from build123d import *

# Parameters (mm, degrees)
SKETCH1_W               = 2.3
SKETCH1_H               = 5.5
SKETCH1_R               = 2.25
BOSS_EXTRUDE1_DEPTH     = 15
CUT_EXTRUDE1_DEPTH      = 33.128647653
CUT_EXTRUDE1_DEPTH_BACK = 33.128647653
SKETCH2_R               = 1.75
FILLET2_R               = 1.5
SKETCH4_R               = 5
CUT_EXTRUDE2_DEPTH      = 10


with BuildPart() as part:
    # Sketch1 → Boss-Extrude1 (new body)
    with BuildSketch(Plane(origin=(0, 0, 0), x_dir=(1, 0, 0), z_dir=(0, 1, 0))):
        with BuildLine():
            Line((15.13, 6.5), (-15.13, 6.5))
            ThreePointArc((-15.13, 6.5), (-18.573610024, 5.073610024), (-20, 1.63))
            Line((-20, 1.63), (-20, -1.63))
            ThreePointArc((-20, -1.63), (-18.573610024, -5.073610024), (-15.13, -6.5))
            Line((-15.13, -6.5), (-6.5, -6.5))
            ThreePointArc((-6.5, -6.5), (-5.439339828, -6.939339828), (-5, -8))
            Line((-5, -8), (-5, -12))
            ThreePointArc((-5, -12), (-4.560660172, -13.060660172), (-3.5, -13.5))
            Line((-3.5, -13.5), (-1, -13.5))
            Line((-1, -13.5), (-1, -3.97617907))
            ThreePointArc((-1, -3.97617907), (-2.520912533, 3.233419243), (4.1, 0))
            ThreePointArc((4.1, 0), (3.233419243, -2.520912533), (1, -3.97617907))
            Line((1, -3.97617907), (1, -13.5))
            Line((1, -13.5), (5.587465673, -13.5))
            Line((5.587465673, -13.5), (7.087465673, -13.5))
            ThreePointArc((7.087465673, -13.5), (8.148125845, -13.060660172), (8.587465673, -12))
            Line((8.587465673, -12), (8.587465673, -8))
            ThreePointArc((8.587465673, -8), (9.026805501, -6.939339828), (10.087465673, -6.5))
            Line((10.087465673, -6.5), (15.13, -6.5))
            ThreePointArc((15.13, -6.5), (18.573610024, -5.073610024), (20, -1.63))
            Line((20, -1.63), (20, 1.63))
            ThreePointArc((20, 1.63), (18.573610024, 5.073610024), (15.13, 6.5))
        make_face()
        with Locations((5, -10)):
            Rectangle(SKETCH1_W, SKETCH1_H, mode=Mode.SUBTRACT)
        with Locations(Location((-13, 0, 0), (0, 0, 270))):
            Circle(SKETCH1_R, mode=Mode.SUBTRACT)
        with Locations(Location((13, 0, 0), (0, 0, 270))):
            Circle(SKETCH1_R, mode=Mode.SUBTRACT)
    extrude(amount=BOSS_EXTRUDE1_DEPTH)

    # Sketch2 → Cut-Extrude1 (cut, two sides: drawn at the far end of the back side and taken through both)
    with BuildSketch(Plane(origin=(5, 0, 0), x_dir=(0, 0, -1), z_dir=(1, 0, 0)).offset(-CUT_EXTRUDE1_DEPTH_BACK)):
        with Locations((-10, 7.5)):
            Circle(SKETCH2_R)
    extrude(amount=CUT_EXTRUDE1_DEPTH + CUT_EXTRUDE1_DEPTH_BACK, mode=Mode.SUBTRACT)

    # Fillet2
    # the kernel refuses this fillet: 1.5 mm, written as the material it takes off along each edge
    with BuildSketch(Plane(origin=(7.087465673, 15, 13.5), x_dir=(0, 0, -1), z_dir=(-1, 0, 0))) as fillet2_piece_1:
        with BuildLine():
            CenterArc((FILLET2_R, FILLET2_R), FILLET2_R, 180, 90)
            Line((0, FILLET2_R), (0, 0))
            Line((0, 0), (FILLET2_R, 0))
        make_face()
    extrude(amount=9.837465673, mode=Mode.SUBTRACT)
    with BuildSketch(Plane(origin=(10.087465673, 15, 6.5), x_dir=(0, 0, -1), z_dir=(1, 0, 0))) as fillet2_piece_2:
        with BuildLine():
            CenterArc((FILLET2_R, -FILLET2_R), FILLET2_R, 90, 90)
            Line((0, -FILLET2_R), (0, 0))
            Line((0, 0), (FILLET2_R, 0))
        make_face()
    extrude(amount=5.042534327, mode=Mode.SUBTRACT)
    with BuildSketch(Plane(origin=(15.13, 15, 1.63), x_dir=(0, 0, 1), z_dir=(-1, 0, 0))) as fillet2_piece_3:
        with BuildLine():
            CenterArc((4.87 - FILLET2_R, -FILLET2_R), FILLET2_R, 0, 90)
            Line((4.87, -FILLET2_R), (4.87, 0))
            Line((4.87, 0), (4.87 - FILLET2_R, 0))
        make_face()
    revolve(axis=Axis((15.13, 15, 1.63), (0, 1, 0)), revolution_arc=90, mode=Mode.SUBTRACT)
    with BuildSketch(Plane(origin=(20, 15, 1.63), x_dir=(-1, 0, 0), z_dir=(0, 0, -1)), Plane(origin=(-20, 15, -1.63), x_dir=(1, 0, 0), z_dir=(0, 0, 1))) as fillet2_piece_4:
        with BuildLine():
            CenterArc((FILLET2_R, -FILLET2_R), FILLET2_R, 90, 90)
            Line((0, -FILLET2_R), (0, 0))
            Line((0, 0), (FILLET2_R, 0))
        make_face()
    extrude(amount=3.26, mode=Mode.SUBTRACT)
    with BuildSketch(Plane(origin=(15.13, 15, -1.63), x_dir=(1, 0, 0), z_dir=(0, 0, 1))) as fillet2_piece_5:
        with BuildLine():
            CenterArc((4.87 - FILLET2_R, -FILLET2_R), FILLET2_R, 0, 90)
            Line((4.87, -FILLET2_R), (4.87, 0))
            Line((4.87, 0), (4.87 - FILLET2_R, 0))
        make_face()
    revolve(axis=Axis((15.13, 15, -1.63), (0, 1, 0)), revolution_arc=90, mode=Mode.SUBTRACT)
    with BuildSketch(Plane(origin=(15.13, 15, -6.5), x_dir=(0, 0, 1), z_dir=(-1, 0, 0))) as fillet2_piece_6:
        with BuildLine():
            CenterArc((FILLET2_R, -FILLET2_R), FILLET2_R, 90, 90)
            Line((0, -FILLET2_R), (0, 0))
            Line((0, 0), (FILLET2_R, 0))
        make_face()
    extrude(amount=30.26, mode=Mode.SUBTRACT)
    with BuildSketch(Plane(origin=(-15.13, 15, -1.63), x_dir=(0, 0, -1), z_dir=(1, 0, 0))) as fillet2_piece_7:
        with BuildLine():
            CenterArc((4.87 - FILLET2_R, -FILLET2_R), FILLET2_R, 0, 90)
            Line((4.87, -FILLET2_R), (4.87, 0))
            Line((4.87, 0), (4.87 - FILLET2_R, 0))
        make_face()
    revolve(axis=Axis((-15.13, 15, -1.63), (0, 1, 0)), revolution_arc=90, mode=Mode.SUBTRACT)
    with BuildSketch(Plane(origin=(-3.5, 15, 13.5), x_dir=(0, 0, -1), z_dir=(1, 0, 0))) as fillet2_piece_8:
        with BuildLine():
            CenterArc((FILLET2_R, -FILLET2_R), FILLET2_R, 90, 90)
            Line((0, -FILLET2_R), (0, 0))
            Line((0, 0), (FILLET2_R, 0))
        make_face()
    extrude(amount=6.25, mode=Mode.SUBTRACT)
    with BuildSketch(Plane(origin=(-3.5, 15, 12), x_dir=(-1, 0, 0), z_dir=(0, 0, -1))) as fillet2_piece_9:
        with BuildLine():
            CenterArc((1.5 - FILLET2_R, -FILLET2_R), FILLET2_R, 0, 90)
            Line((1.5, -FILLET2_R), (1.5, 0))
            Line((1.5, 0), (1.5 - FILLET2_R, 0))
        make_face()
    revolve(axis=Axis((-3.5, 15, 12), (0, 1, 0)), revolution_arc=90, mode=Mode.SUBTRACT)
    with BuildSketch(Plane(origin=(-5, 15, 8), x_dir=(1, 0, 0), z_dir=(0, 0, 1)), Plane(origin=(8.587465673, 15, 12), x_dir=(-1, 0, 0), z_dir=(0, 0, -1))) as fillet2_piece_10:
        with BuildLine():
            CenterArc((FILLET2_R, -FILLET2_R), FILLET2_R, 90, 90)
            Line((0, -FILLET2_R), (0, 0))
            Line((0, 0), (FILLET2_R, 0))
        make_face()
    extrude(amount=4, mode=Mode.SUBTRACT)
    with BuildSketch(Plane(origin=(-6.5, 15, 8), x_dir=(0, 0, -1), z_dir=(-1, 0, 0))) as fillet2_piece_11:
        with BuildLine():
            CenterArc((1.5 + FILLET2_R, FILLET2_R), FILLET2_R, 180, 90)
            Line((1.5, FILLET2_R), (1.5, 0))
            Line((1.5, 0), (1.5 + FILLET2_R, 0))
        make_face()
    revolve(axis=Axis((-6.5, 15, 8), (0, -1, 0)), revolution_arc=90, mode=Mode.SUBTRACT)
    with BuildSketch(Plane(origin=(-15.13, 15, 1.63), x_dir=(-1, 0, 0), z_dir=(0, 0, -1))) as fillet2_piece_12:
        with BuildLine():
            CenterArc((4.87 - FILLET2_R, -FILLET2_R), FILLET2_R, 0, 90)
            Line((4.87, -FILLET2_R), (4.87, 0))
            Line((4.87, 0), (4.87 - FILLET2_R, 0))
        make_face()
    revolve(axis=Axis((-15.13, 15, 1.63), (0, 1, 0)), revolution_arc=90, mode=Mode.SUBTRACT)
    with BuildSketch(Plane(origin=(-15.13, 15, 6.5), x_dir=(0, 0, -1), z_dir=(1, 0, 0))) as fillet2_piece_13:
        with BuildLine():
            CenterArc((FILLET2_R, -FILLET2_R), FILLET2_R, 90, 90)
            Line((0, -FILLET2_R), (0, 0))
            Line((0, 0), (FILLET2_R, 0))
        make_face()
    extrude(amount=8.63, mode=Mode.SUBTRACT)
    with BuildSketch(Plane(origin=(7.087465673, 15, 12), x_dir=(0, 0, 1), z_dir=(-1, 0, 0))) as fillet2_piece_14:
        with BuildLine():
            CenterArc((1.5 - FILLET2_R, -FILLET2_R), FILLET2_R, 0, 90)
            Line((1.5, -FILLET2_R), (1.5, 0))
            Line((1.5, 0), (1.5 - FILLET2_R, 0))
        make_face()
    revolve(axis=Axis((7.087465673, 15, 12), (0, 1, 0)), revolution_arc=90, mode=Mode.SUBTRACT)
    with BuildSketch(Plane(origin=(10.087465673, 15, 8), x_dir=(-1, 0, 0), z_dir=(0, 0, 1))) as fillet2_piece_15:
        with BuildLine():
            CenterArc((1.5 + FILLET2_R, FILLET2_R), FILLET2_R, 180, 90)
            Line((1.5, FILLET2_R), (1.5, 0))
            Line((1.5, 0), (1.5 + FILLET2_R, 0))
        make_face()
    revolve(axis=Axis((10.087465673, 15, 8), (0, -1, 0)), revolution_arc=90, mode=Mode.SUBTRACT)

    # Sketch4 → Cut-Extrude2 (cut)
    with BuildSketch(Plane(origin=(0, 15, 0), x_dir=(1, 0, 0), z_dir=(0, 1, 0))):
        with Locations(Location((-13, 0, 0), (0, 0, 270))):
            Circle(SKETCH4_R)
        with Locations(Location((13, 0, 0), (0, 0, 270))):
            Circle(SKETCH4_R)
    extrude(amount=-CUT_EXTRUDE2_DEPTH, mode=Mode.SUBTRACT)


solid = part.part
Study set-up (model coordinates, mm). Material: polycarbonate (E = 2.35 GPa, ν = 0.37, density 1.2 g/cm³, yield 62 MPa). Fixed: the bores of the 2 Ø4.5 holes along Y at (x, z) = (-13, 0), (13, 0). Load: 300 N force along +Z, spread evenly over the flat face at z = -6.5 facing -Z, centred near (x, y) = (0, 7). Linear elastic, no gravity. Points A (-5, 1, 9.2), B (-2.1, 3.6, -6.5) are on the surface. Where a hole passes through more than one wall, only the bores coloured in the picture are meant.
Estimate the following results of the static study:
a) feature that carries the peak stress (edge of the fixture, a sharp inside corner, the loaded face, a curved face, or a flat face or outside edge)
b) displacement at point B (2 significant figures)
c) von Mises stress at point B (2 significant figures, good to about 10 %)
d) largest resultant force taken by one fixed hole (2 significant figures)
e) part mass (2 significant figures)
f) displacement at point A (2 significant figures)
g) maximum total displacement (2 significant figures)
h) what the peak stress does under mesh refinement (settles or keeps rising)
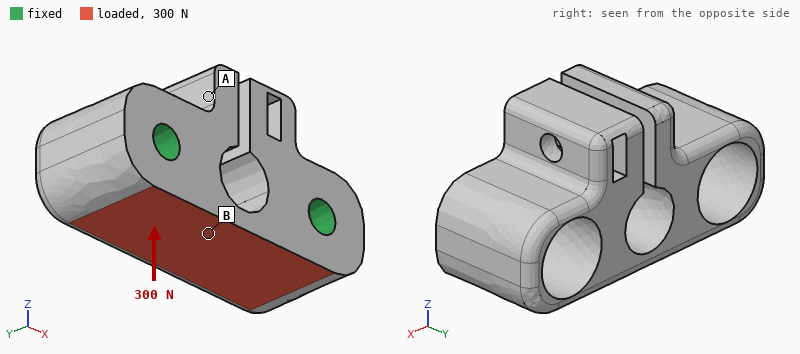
edge of the fixture
40 µm
3.1 MPa
160 N
6.9 g
38 µm
89 µm
keeps rising
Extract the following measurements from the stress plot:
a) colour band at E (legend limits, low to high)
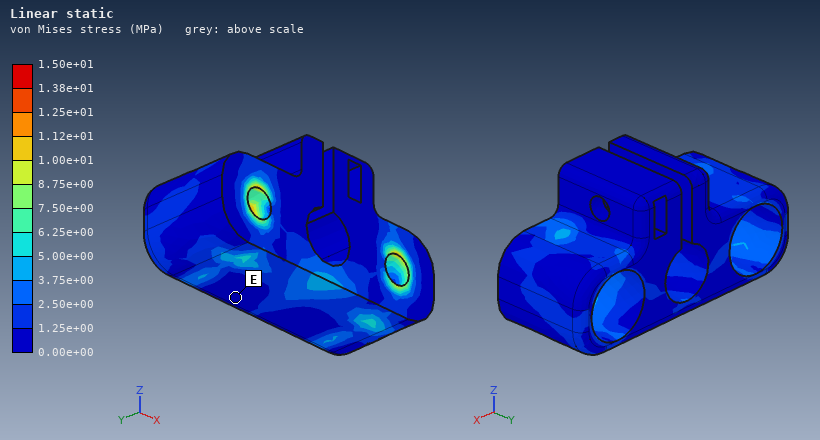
0.00e+00 to 1.25e+00 MPa
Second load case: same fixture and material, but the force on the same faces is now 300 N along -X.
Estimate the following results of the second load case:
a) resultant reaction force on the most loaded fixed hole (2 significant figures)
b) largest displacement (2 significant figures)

160 N
28 µm
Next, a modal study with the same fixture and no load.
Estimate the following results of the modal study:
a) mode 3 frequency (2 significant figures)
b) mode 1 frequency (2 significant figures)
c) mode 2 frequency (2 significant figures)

4600 Hz
4000 Hz
4300 Hz
